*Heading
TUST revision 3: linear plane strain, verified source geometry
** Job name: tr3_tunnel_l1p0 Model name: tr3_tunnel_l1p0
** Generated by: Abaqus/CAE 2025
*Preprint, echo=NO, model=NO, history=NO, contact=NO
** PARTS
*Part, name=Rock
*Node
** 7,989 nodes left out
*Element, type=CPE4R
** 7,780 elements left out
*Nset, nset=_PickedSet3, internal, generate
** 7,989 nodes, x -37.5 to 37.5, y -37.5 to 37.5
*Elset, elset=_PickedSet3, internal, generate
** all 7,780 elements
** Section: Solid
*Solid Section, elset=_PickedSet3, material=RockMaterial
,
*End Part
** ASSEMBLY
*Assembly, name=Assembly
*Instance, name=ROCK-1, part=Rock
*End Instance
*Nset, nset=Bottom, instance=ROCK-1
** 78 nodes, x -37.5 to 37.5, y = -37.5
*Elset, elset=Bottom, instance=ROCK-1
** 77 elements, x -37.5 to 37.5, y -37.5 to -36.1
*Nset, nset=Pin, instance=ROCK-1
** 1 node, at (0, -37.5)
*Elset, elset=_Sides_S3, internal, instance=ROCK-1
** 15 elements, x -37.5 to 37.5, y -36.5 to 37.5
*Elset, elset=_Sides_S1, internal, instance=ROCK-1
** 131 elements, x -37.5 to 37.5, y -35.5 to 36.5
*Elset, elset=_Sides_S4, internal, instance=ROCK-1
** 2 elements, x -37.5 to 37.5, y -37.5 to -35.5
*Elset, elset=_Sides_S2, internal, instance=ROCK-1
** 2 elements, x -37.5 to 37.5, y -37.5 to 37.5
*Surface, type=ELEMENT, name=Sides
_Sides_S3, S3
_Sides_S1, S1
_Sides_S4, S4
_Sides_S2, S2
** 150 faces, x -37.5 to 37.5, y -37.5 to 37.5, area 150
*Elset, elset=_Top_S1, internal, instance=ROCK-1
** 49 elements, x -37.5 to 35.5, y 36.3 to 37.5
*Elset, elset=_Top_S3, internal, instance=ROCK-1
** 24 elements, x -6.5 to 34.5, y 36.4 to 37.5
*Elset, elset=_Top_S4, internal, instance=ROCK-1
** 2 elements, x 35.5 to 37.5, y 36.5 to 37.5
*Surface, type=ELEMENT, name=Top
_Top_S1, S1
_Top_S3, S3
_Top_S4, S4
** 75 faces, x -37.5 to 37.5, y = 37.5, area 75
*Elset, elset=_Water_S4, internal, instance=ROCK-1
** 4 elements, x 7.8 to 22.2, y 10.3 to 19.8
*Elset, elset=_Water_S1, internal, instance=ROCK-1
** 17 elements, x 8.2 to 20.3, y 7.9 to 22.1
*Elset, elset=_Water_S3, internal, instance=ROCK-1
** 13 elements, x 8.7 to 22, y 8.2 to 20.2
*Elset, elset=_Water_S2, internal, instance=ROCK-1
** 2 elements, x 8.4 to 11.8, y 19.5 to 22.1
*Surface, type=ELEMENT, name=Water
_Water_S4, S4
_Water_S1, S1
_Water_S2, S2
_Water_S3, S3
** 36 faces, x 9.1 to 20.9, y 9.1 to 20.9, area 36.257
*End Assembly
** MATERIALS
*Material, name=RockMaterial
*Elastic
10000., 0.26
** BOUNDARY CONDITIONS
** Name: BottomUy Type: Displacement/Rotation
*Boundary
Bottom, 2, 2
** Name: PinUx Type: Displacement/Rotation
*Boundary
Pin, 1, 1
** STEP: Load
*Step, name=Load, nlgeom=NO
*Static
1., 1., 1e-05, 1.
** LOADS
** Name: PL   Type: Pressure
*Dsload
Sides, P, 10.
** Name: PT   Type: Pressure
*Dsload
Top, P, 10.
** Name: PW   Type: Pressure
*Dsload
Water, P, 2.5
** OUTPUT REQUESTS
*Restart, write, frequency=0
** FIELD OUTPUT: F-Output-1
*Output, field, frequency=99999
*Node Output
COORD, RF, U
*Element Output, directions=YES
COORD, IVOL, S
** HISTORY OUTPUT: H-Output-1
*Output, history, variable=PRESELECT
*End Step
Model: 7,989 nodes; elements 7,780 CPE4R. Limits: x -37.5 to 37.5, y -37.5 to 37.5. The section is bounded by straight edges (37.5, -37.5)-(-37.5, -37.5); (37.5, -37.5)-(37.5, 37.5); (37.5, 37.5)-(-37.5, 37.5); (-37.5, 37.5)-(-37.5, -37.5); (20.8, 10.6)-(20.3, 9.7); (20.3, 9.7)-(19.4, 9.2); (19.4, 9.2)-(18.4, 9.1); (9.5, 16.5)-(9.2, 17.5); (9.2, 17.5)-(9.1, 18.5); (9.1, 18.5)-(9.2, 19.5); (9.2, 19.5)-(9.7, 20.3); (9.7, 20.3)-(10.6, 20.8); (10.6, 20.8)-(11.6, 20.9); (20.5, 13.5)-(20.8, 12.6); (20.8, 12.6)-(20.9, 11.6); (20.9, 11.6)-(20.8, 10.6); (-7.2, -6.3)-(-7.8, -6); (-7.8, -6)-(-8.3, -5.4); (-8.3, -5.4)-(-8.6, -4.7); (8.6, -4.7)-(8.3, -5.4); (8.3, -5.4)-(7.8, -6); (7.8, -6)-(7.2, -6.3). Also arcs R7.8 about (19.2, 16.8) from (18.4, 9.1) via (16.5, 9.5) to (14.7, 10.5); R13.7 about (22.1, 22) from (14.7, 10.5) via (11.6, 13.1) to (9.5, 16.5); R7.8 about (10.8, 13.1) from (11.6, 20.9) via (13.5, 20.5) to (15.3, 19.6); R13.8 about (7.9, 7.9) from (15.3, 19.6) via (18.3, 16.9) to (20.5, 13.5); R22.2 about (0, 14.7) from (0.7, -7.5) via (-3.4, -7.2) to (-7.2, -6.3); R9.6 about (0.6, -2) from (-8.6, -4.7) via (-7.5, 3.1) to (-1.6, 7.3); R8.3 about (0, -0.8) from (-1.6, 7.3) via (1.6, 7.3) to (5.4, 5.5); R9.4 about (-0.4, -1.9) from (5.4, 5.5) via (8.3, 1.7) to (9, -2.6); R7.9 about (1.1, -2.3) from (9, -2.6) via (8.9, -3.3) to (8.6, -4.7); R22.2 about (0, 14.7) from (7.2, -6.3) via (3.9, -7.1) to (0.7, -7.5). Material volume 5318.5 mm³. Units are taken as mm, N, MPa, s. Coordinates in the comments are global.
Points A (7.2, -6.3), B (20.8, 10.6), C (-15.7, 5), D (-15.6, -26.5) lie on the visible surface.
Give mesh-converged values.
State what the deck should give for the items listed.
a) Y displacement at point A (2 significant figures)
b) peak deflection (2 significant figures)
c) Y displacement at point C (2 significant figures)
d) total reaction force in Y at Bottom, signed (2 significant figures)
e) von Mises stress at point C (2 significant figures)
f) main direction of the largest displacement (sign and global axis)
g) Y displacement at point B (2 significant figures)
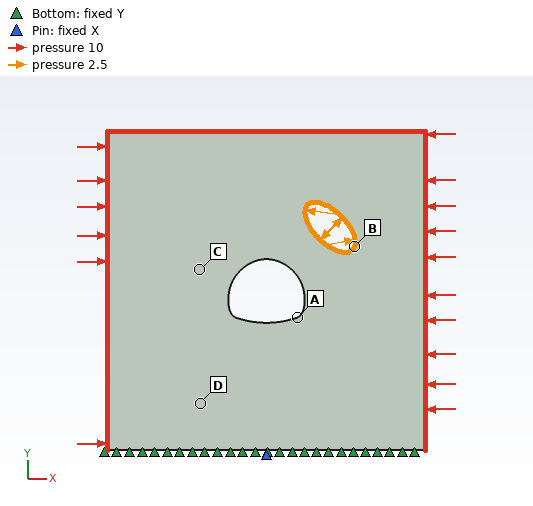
-0.013 mm
0.061 mm
-0.032 mm
750 N
7.3 MPa
-Y
-0.035 mm
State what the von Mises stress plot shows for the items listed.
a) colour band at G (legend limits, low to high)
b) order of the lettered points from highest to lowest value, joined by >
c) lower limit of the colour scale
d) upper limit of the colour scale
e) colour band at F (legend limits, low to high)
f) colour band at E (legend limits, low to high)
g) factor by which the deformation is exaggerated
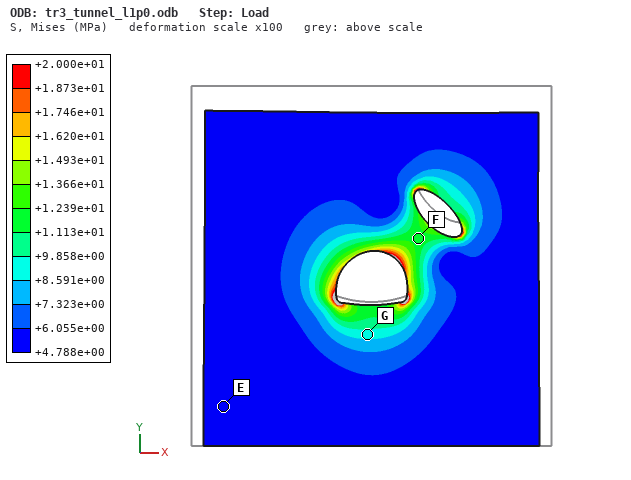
+8.591e+00 to +9.858e+00 MPa
F > G > E
+4.788e+00 MPa
+2.000e+01 MPa
+1.113e+01 to +1.239e+01 MPa
+4.788e+00 to +6.055e+00 MPa
100
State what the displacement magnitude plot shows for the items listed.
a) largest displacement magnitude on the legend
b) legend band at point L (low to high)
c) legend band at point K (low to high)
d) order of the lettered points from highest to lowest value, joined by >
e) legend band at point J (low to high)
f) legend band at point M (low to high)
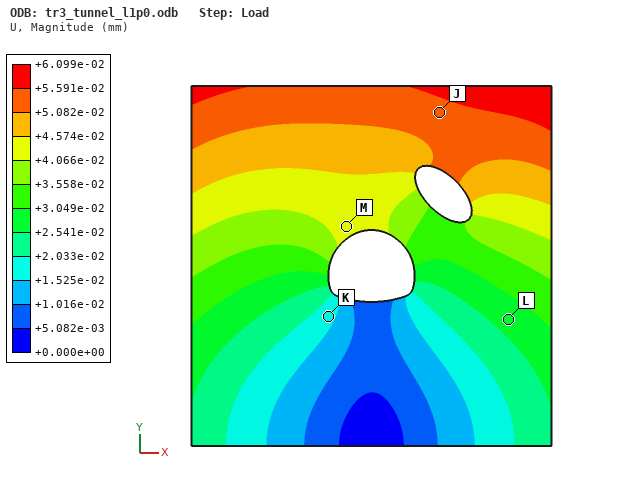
+6.099e-02 mm
+2.541e-02 to +3.049e-02 mm
+1.525e-02 to +2.033e-02 mm
J > M > L > K
+5.082e-02 to +5.591e-02 mm
+4.066e-02 to +4.574e-02 mm
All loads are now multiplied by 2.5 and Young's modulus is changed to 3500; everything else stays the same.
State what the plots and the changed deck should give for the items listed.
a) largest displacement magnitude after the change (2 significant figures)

0.44 mm
